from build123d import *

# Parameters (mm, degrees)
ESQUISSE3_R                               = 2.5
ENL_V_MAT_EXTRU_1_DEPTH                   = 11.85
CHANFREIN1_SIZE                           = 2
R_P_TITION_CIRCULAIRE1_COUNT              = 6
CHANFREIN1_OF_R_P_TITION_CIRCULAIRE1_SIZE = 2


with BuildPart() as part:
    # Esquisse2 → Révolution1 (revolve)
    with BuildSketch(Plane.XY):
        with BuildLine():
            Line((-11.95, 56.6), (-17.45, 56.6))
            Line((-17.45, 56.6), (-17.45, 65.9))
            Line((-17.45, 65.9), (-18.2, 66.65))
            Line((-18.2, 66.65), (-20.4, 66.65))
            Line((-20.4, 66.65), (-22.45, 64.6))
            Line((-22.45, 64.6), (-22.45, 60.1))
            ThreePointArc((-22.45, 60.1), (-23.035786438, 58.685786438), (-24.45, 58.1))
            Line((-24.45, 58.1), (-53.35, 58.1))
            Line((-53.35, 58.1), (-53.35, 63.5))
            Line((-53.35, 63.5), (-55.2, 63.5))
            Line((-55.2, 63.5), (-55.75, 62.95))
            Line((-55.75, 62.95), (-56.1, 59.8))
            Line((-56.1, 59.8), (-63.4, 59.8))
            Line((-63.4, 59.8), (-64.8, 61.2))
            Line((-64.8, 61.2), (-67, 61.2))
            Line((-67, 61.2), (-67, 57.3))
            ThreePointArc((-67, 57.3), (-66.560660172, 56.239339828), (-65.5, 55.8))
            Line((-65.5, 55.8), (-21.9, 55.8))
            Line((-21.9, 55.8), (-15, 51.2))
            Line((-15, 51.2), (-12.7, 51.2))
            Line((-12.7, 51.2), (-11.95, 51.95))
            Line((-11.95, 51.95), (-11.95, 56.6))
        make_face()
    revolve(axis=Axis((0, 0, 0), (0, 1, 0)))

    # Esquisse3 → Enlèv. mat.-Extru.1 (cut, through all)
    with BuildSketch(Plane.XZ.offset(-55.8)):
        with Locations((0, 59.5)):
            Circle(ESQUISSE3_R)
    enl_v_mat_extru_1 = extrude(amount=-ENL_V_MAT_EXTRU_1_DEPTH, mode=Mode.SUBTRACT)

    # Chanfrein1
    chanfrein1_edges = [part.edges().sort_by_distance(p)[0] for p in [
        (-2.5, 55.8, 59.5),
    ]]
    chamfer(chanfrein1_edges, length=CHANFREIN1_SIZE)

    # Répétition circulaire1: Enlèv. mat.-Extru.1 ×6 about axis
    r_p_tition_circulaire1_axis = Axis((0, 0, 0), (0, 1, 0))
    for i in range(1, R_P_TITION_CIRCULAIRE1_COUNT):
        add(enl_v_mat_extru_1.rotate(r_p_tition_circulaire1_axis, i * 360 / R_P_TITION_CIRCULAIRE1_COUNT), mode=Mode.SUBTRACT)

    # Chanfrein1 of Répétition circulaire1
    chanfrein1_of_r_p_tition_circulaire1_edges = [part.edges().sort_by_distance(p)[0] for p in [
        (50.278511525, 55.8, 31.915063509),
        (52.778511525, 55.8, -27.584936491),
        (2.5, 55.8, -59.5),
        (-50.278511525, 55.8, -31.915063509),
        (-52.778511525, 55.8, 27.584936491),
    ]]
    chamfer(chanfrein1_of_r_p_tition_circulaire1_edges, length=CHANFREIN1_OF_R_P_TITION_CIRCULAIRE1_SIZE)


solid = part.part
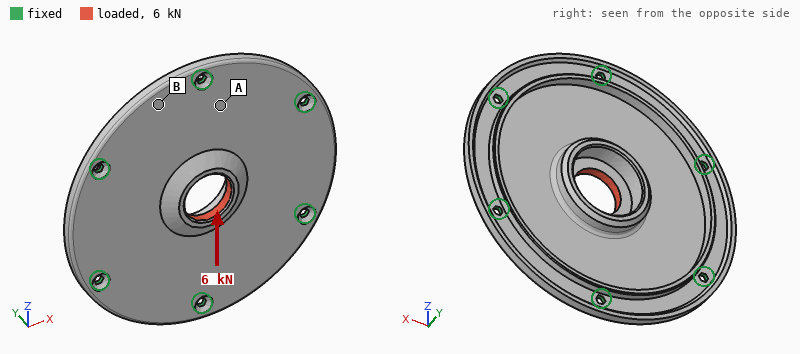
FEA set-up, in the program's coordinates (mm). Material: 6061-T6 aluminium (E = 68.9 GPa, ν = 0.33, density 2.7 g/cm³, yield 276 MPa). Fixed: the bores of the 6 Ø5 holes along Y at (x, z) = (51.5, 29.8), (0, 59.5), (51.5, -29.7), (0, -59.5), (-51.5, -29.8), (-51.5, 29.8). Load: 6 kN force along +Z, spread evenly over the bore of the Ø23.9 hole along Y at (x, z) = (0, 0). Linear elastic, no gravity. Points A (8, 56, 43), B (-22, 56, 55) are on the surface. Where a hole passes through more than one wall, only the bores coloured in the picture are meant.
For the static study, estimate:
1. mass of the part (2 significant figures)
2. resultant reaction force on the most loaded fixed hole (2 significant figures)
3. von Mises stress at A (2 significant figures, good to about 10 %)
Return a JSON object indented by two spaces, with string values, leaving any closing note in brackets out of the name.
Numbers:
{
  "mass of the part": "140 g",
  "resultant reaction force on the most loaded fixed hole": "1.4 kN",
  "von Mises stress at A": "14 MPa"
}
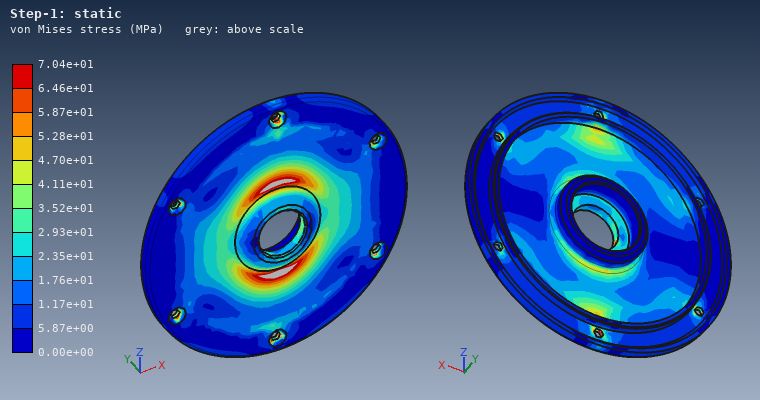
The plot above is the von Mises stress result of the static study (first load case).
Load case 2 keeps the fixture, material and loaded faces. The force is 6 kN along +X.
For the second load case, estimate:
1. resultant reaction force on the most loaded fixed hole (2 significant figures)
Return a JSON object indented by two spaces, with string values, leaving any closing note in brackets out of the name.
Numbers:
{
  "resultant reaction force on the most loaded fixed hole": "1.2 kN"
}
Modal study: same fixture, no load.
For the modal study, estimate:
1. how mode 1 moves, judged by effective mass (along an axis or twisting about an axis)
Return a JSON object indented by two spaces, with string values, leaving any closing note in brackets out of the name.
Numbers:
{
  "how mode 1 moves, judged by effective mass": "along Y"
}
